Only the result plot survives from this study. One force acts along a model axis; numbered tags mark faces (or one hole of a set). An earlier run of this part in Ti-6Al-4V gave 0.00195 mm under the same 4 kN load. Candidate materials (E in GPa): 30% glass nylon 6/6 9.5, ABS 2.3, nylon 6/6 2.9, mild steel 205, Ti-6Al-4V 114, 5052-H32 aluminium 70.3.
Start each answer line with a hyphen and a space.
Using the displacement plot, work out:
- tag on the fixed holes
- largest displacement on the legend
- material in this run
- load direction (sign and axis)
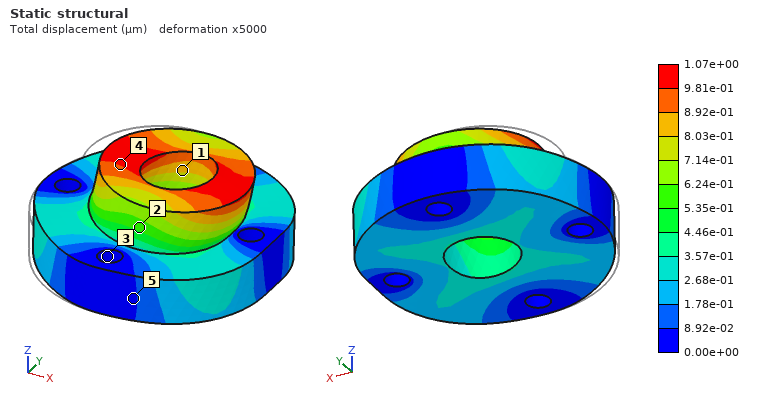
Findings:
- 3
- 1.07e+00 µm
- mild steel
- +X
